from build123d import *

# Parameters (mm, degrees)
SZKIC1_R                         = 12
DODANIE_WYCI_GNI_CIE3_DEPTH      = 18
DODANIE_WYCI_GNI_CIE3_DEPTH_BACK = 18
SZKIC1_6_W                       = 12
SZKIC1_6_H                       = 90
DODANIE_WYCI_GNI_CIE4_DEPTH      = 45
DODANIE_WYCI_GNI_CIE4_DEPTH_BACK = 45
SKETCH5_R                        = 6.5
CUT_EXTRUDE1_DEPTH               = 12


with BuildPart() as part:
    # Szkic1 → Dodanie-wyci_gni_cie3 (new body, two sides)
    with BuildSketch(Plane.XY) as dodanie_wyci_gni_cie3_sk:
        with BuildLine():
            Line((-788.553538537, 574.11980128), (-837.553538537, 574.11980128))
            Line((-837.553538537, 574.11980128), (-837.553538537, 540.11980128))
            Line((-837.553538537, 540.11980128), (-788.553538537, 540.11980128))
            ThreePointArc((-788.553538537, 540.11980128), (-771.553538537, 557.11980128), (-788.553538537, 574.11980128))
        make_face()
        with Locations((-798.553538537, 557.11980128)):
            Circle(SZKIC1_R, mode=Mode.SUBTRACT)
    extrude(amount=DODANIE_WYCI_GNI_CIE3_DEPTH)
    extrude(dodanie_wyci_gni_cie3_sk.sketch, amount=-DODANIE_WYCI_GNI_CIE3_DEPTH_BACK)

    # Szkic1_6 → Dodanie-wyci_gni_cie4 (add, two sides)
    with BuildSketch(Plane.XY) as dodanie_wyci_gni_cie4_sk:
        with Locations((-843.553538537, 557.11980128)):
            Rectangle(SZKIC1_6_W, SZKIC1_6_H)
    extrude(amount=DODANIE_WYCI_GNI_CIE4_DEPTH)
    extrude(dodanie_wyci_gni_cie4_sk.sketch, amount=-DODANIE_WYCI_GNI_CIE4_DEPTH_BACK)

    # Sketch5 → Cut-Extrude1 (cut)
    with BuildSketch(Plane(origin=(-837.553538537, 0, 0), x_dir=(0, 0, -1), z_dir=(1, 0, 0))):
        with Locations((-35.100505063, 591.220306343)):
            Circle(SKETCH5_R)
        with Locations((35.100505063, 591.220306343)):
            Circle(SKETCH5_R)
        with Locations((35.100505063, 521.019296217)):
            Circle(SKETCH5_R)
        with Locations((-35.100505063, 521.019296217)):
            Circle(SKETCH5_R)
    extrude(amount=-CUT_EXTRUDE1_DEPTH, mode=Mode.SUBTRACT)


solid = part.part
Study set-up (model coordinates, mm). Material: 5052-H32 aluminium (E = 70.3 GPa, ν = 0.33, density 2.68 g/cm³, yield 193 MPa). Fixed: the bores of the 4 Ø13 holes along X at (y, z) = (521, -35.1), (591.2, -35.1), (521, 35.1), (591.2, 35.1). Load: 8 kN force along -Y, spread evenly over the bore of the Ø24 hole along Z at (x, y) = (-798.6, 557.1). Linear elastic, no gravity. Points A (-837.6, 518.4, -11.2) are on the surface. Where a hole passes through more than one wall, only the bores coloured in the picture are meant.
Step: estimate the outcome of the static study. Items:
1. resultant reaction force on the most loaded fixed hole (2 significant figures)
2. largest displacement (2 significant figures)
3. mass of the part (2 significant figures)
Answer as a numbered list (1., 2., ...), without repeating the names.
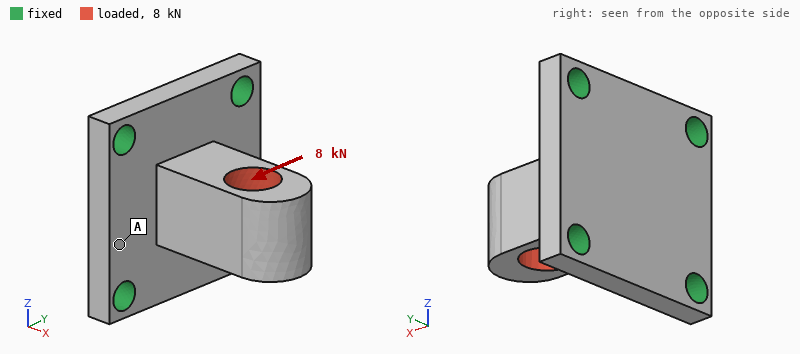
1. 3.9 kN
2. 0.19 mm
3. 400 g
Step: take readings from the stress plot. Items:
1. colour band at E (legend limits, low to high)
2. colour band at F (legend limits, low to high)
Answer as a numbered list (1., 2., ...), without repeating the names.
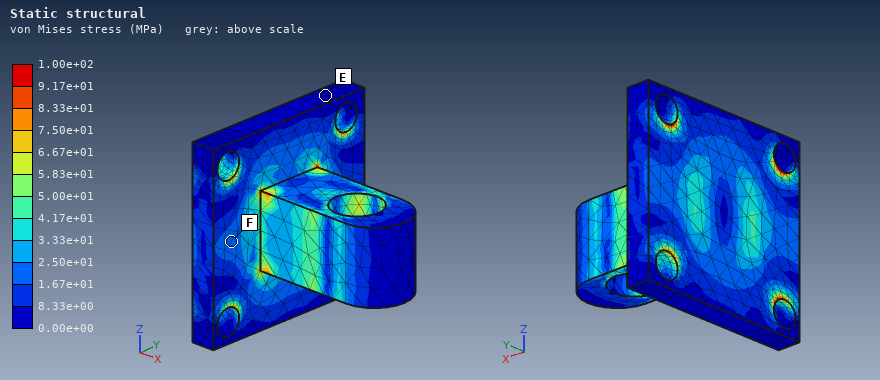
1. 0.00e+00 to 8.33e+00 MPa
2. 1.67e+01 to 2.50e+01 MPa
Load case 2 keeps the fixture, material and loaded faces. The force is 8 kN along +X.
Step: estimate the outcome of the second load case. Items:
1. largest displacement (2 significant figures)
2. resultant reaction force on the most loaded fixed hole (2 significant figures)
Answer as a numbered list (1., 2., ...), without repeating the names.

1. 28 µm
2. 2.1 kN
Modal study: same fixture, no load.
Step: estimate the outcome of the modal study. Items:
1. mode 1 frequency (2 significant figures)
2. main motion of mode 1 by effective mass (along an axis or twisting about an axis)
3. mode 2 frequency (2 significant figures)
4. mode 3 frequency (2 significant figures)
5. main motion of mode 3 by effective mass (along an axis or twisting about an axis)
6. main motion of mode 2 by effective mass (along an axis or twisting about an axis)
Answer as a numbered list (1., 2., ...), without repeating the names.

1. 3500 Hz
2. along Y
3. 3900 Hz
4. 6300 Hz
5. along X
6. along Z
